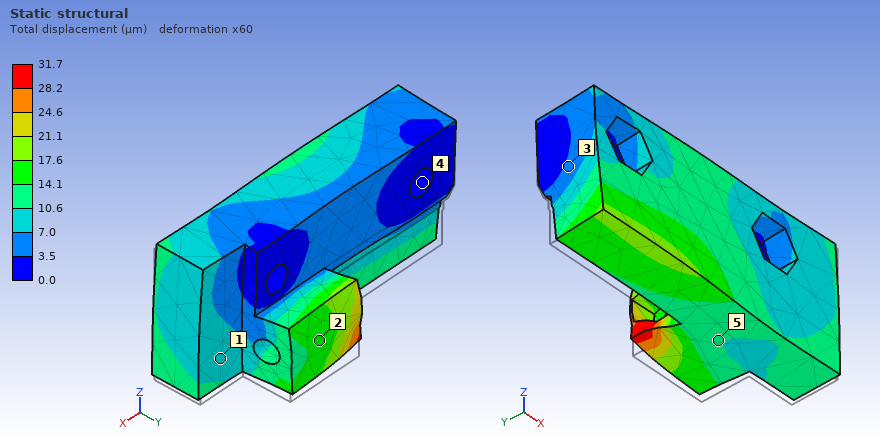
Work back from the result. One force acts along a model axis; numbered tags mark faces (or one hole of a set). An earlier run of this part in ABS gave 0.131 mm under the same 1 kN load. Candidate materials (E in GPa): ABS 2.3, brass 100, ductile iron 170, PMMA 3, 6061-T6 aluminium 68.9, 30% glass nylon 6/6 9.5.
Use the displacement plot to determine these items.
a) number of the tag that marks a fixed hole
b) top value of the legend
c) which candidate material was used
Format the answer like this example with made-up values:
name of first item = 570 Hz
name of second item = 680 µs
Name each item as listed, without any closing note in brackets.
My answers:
number of the tag that marks a fixed hole = 4
top value of the legend = 31.7 µm
which candidate material was used = 30% glass nylon 6/6
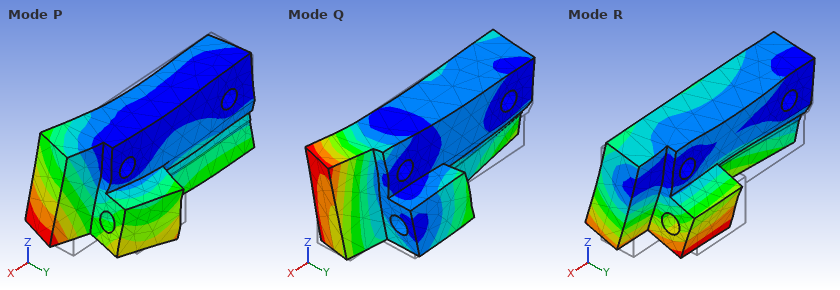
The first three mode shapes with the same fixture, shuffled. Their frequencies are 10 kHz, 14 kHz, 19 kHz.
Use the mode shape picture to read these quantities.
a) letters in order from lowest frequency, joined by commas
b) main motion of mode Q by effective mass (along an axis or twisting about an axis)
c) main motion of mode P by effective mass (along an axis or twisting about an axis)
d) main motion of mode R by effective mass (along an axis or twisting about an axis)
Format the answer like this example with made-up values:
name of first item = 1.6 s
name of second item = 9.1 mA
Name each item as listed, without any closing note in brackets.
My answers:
letters in order from lowest frequency, joined by commas = R, P, Q
main motion of mode Q by effective mass = along X
main motion of mode P by effective mass = twisting about Z
main motion of mode R by effective mass = along Y
